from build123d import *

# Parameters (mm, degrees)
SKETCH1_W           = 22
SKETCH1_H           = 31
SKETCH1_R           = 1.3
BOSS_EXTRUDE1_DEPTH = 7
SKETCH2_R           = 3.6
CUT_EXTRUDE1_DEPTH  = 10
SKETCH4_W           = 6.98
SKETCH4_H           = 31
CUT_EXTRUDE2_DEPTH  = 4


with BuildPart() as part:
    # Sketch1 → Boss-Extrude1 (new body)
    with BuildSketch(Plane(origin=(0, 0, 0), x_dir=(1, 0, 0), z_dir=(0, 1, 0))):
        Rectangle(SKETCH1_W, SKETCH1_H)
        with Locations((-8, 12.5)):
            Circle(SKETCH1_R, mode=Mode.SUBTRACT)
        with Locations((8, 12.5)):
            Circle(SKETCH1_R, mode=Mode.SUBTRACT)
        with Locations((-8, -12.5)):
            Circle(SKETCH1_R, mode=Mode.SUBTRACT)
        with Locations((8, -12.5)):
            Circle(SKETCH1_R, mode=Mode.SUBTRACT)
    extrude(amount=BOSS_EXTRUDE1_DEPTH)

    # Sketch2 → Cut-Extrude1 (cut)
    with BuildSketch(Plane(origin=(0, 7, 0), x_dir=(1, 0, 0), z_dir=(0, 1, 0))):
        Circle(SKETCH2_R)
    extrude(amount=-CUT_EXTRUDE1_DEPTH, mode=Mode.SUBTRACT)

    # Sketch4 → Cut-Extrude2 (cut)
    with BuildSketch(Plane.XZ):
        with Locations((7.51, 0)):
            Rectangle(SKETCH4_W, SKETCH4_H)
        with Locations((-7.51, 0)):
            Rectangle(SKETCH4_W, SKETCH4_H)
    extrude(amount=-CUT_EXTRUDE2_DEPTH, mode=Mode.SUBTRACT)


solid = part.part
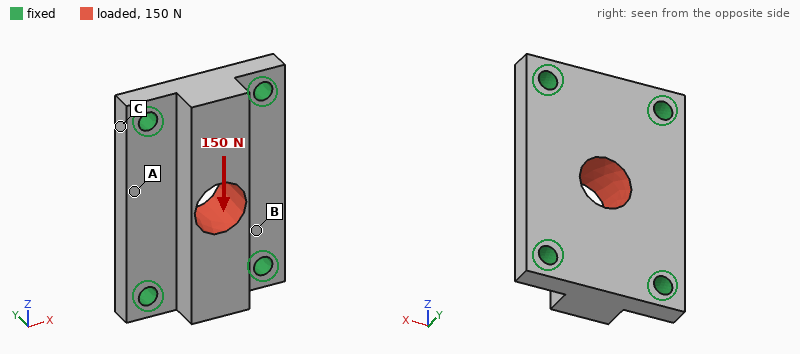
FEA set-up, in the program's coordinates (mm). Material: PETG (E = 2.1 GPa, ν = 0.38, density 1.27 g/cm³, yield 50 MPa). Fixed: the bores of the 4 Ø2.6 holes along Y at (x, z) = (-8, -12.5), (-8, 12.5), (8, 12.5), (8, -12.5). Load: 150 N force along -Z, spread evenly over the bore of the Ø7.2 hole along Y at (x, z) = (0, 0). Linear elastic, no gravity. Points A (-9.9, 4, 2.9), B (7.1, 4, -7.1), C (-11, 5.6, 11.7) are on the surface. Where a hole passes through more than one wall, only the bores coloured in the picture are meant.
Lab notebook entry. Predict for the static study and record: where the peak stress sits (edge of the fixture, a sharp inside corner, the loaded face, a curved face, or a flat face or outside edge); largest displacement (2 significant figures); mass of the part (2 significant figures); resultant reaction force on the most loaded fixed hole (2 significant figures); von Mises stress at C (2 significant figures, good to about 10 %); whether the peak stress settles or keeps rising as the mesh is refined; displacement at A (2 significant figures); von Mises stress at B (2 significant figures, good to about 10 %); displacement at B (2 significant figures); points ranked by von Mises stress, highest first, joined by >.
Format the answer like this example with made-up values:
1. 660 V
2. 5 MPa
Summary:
1. edge of the fixture
2. 14 µm
3. 3.4 g
4. 40 N
5. 0.85 MPa
6. keeps rising
7. 3.6 µm
8. 1.6 MPa
9. 3.8 µm
10. B > C > A
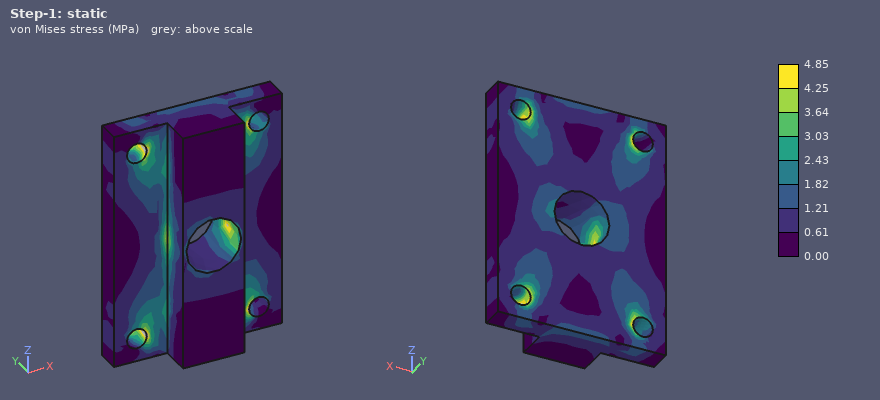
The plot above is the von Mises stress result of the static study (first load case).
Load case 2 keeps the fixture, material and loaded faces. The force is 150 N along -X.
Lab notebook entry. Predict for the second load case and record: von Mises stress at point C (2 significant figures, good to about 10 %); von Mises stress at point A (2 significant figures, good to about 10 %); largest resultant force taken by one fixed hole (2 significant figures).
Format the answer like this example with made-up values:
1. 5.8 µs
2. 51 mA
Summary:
1. 1.9 MPa
2. 0.75 MPa
3. 47 N
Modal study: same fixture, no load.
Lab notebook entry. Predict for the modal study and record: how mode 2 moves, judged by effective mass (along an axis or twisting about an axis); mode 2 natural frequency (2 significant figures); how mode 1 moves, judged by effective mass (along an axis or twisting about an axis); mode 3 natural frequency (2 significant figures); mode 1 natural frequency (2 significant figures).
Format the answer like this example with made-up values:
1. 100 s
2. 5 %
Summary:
1. twisting about Z
2. 8600 Hz
3. along Y
4. 11 kHz
5. 5800 Hz
